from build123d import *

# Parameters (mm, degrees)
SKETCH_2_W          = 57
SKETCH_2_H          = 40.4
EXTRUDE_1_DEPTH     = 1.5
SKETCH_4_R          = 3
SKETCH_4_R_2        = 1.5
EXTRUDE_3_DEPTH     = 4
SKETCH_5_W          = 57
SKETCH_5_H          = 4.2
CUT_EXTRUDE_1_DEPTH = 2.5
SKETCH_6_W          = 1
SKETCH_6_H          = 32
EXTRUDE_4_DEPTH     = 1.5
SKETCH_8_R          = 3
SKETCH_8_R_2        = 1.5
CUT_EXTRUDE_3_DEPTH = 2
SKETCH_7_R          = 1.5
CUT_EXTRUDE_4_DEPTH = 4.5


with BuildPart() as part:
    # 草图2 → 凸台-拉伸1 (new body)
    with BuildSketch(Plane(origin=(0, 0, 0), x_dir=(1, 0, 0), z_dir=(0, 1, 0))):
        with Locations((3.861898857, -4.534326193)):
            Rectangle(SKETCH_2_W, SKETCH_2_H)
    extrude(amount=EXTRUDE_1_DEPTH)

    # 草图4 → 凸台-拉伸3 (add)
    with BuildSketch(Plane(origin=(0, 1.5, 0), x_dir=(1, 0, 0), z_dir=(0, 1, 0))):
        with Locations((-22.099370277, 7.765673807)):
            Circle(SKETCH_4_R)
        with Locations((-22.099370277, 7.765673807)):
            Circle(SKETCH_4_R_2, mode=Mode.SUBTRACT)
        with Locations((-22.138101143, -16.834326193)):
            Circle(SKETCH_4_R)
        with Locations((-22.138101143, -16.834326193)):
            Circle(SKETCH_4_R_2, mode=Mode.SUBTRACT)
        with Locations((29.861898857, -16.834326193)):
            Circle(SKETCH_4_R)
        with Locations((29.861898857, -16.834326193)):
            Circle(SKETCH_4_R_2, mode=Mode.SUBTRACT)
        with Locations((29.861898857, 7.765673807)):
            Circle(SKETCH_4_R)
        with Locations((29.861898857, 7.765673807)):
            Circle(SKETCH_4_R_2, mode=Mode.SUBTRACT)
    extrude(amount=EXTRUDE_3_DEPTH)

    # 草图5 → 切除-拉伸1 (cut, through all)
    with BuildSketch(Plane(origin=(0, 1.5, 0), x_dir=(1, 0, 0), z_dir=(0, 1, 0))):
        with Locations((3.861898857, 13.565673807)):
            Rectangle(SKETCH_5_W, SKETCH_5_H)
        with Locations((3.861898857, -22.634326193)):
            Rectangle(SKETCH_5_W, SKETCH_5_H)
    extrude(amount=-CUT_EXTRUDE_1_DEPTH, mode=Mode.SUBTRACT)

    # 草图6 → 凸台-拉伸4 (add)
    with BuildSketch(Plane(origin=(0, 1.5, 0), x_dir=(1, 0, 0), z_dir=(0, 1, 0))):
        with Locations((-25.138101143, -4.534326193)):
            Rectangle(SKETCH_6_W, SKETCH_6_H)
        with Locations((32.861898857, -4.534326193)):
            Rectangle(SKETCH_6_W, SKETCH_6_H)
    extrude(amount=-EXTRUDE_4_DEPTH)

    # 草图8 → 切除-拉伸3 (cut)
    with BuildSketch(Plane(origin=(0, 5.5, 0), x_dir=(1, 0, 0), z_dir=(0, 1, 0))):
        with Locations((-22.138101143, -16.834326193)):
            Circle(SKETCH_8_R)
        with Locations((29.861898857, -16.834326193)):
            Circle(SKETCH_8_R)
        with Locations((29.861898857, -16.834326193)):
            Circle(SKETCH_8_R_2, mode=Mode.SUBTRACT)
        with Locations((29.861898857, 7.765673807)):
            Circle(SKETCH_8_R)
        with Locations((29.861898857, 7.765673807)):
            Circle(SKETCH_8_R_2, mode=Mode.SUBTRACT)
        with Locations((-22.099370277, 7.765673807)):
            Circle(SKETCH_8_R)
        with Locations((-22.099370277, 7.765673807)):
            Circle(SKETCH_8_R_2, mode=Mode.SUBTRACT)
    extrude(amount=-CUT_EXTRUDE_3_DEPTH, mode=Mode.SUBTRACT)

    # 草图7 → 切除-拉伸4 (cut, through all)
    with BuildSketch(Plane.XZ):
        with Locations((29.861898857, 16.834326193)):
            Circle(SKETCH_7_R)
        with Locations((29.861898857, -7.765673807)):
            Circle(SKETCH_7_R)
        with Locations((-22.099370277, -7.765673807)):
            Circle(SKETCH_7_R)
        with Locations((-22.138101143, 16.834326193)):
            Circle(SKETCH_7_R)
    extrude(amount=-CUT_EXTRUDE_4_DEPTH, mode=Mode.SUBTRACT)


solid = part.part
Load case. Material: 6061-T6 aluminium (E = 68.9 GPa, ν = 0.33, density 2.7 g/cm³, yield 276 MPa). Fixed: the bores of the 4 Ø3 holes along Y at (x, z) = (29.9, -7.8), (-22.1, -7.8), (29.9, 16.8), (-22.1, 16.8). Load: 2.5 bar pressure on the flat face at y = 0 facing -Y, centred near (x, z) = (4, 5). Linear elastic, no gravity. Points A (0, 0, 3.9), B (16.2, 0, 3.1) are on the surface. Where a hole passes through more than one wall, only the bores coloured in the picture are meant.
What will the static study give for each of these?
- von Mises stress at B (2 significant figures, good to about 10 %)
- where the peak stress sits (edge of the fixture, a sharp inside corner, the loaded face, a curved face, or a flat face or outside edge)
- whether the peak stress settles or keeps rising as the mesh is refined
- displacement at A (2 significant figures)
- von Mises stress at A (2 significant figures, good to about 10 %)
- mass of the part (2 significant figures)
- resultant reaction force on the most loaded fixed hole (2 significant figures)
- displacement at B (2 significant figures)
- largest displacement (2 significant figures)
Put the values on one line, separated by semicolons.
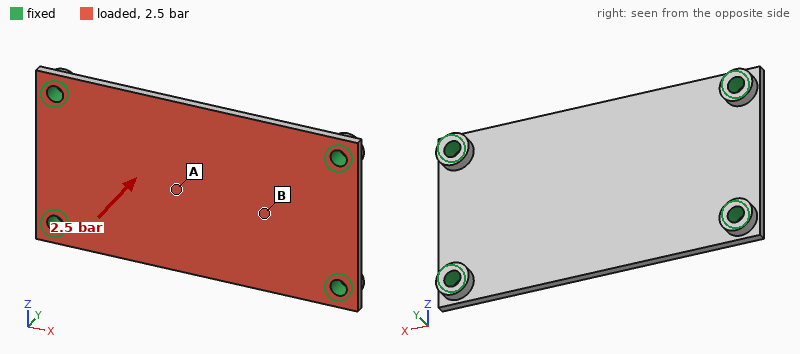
23 MPa; edge of the fixture; keeps rising; 0.21 mm; 58 MPa; 8.0 g; 120 N; 0.14 mm; 0.22 mm
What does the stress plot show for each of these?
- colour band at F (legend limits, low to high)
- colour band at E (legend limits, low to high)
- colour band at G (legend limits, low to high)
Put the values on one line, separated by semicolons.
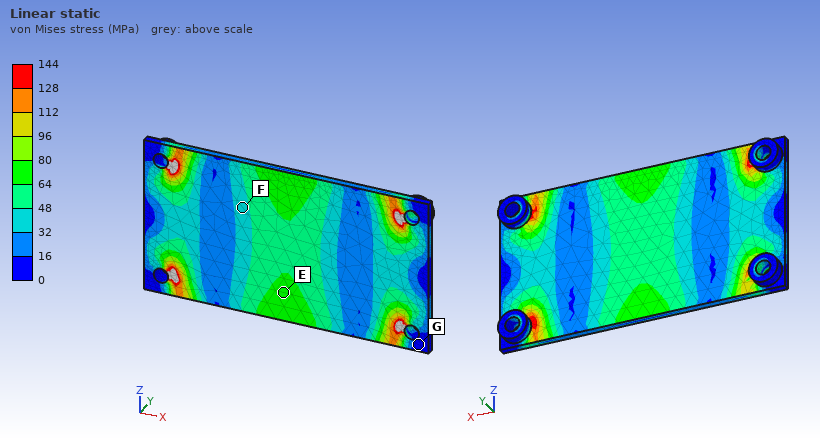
32 to 48 MPa; 64 to 80 MPa; 0 to 16 MPa
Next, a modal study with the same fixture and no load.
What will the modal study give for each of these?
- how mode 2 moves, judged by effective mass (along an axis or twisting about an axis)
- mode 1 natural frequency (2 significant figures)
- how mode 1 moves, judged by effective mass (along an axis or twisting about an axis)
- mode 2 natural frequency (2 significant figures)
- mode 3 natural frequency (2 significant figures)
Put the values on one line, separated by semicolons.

twisting about X; 3100 Hz; along Y; 4700 Hz; 8200 Hz
